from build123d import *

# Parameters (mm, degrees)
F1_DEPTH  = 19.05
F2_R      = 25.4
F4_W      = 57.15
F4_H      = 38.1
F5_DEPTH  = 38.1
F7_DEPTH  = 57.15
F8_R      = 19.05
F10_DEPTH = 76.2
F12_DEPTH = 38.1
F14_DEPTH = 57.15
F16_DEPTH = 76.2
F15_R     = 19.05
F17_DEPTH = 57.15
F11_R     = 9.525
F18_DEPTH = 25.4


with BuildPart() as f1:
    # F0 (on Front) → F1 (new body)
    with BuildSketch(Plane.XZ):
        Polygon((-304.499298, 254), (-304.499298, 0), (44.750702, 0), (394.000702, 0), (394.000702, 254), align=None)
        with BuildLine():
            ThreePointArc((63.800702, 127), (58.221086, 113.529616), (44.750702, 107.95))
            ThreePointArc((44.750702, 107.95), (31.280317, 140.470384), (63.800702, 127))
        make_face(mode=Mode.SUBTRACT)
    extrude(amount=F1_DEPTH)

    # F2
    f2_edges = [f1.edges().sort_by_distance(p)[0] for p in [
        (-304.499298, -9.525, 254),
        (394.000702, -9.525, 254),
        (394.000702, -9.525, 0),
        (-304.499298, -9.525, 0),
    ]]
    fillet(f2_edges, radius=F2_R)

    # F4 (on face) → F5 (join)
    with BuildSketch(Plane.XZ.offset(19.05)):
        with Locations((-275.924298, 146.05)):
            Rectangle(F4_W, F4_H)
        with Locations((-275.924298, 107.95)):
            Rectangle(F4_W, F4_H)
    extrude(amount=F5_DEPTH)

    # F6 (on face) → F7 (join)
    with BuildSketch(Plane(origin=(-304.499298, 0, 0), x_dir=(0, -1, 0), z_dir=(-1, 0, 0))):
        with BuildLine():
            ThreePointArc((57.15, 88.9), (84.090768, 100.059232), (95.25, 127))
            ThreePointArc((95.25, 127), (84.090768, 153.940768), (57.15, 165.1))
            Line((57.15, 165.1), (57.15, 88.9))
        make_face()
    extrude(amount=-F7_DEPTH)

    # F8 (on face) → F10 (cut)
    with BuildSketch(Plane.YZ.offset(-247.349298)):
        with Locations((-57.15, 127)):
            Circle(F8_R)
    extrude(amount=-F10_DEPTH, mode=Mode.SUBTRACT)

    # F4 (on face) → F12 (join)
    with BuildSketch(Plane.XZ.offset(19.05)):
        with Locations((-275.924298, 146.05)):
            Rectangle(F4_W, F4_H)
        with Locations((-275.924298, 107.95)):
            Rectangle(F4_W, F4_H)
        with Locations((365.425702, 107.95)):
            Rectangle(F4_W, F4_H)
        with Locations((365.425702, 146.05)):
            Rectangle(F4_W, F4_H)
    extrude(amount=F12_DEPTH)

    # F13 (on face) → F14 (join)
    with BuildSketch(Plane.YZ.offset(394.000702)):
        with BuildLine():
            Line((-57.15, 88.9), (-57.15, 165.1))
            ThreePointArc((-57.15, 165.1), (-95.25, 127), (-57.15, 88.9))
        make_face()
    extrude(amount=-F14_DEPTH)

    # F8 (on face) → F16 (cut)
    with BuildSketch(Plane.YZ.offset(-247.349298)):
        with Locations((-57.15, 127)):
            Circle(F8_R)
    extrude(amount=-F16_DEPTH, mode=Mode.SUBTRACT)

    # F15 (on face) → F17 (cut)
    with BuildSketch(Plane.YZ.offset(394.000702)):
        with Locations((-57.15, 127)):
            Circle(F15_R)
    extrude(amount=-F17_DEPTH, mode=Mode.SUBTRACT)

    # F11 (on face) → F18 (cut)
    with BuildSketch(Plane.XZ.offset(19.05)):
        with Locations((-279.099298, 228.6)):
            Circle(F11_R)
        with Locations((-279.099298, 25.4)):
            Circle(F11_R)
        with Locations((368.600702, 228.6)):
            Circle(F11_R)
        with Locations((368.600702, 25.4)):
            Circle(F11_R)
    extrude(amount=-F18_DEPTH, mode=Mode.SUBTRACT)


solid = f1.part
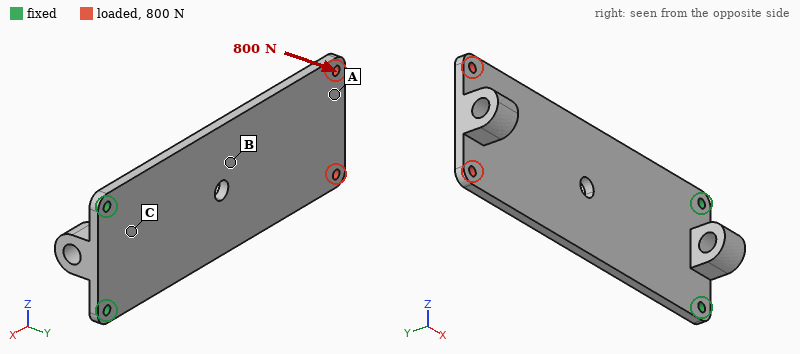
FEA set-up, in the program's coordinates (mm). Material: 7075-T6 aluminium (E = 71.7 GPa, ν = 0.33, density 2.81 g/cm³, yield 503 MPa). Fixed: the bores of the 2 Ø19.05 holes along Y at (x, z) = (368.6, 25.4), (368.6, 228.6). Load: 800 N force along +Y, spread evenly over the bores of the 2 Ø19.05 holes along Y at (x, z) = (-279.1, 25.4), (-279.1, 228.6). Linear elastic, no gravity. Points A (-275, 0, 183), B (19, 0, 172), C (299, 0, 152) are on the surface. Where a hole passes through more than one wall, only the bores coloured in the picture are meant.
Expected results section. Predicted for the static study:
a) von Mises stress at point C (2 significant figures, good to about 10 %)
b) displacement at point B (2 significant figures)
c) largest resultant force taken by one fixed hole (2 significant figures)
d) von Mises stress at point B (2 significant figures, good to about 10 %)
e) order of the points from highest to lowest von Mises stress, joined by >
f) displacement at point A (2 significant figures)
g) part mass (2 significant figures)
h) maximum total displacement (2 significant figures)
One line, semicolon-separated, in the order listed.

27 MPa; 2.7 mm; 400 N; 17 MPa; C > B > A; 7.4 mm; 11 kg; 8.0 mm
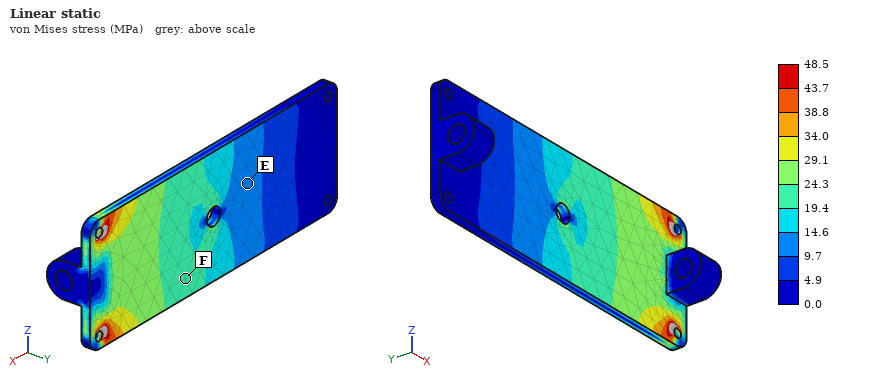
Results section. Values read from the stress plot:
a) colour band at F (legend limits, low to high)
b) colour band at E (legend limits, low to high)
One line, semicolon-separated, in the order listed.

19.4 to 24.3 MPa; 9.7 to 14.6 MPa
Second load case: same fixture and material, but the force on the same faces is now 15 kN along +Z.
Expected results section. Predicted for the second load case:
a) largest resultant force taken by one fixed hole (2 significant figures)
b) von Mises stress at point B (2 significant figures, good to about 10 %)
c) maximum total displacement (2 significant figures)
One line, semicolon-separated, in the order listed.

48 kN; 9.7 MPa; 0.91 mm
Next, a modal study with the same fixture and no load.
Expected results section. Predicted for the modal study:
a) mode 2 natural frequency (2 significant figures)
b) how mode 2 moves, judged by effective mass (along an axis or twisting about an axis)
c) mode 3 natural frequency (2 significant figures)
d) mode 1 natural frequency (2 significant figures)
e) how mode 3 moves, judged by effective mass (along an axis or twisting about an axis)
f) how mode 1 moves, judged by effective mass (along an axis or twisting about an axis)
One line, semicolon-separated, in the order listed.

180 Hz; twisting about X; 190 Hz; 30 Hz; along Y; along Y
